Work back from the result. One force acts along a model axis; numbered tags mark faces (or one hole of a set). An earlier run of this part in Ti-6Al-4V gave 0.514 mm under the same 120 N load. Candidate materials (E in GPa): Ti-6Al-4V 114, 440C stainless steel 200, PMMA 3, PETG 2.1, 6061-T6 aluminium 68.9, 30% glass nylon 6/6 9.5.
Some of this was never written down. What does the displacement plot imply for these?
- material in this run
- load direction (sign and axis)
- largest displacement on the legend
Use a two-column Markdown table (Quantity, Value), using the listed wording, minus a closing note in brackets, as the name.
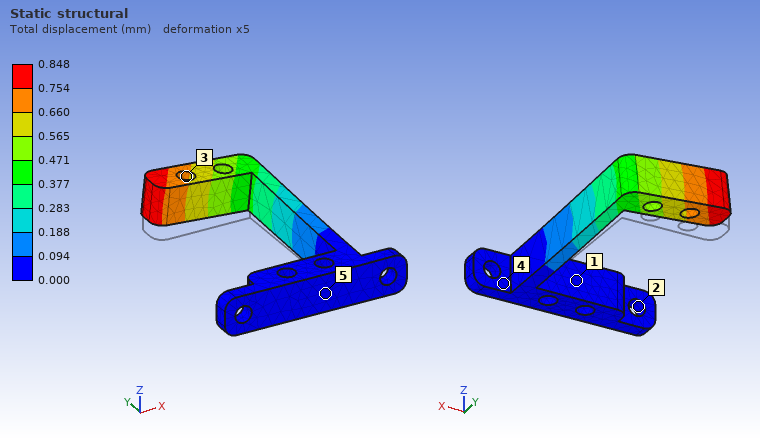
| Quantity | Value |
|---|---|
| material in this run | 6061-T6 aluminium |
| load direction | +Z |
| largest displacement on the legend | 0.848 mm |
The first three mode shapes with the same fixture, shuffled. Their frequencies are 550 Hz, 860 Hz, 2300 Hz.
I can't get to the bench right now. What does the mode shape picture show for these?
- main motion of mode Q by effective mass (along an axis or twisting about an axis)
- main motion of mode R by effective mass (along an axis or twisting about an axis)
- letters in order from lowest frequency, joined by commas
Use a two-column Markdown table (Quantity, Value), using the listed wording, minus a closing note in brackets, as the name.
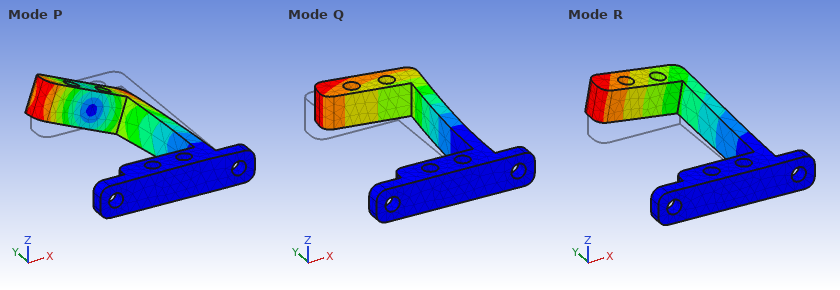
| Quantity | Value |
|---|---|
| main motion of mode Q by effective mass | along X |
| main motion of mode R by effective mass | along Z |
| letters in order from lowest frequency, joined by commas | Q, R, P |
